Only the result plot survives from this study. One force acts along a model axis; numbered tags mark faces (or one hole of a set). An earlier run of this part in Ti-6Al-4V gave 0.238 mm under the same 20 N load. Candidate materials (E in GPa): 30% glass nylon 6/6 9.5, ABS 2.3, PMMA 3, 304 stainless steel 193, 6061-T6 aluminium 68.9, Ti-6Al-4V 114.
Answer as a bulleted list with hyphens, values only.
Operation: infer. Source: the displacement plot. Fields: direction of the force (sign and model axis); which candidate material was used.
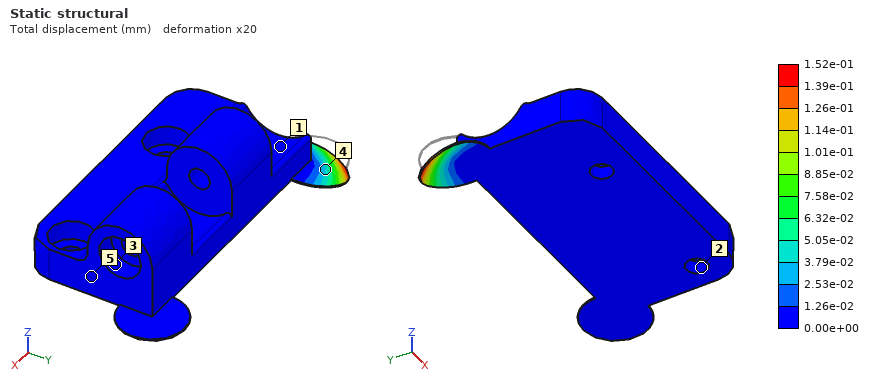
- -Z
- 304 stainless steel
